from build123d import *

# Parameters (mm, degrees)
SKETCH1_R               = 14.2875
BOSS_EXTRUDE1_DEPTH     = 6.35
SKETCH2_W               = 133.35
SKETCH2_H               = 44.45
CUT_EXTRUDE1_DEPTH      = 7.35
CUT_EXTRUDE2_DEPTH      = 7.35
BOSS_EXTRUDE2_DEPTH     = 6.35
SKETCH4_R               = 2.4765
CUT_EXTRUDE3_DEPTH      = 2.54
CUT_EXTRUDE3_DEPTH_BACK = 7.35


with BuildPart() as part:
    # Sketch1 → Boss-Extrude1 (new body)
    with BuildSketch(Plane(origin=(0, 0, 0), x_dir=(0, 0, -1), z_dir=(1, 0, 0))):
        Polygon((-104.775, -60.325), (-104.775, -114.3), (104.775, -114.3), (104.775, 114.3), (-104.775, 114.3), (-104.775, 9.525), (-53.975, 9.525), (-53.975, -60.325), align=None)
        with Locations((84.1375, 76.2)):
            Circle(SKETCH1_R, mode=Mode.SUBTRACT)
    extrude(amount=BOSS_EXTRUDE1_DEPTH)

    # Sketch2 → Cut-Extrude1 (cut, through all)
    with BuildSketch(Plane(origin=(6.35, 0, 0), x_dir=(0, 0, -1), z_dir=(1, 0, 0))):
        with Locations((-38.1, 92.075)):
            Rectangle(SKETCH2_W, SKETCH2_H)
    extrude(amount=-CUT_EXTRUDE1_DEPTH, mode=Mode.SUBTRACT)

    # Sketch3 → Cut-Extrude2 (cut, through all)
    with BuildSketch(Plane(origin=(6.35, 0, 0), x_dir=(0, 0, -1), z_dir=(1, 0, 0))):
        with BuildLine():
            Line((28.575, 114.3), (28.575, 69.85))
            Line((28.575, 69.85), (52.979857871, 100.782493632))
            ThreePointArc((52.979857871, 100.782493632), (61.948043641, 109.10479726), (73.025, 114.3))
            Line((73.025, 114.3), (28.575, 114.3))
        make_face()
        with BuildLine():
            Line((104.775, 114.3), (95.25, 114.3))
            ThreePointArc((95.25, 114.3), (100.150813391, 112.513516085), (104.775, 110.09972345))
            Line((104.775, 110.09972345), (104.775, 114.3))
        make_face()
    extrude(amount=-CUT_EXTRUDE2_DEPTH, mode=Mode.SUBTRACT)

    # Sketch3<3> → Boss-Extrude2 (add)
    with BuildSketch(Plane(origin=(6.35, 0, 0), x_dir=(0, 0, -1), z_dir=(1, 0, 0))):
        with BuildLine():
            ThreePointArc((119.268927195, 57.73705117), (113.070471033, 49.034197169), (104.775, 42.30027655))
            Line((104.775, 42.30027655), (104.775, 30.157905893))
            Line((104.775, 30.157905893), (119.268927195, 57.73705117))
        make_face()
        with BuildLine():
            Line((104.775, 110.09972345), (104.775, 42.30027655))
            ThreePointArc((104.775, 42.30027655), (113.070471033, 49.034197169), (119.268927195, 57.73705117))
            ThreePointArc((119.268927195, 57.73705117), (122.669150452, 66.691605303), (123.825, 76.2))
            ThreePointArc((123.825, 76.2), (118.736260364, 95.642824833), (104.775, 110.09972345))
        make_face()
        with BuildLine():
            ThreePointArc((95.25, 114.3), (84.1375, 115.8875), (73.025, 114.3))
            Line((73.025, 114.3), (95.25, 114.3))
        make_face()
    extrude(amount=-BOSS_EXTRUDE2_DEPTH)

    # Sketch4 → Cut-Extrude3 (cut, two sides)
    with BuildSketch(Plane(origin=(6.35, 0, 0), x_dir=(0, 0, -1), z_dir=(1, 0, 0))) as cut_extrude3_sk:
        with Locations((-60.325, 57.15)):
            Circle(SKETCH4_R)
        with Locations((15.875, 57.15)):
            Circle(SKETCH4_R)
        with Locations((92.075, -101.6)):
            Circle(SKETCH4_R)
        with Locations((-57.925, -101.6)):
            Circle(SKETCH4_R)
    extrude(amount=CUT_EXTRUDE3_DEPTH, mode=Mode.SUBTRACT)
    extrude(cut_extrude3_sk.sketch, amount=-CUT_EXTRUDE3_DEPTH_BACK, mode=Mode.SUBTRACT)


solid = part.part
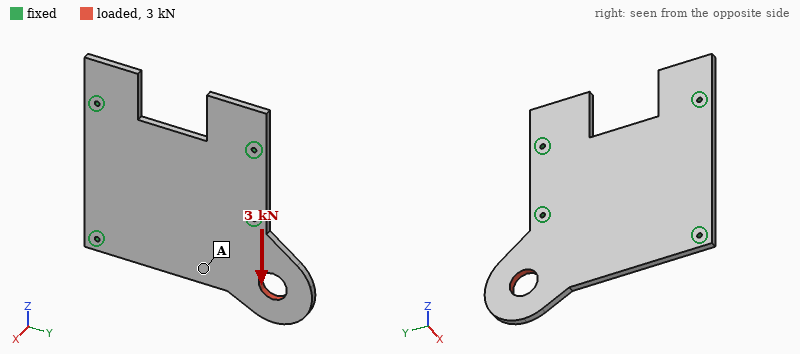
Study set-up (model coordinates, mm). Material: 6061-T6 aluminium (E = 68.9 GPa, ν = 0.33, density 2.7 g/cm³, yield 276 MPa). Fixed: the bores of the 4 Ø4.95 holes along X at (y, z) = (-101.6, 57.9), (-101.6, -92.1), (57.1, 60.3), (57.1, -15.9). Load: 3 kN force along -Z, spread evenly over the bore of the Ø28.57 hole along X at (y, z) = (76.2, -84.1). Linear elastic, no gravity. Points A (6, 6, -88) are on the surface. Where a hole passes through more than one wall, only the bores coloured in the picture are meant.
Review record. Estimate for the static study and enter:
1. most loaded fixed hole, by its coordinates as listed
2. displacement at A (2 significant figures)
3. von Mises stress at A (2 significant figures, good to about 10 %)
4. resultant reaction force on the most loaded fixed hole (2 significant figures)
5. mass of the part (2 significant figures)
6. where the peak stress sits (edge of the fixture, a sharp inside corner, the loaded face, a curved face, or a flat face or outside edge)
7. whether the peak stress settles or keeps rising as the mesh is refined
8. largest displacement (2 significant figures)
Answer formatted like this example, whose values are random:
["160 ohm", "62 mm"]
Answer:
["(57.1, -15.9)", "5.4 µm", "4.0 MPa", "2.7 kN", "650 g", "edge of the fixture", "keeps rising", "32 µm"]
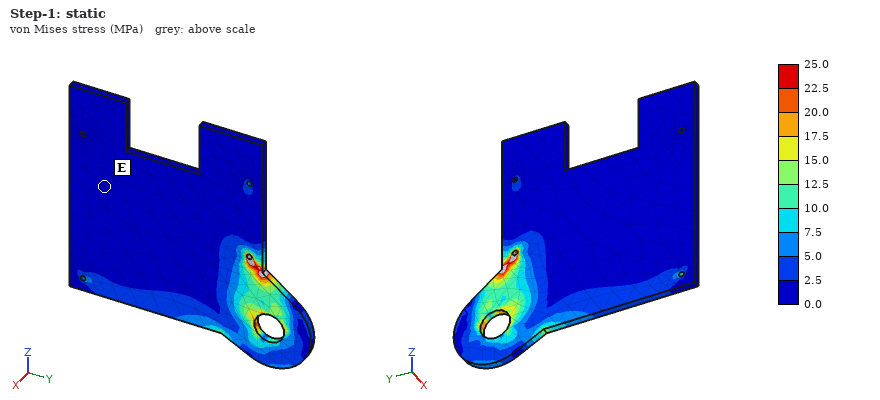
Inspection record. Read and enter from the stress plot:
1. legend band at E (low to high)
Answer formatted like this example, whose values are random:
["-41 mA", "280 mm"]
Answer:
["0.0 to 2.5 MPa"]
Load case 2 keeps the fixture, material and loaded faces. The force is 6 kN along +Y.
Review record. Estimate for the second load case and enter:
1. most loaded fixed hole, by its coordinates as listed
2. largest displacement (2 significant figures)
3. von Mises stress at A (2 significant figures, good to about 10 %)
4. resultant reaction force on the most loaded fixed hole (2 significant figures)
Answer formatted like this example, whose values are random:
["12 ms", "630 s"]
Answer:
["(57.1, -15.9)", "61 µm", "16 MPa", "2.9 kN"]
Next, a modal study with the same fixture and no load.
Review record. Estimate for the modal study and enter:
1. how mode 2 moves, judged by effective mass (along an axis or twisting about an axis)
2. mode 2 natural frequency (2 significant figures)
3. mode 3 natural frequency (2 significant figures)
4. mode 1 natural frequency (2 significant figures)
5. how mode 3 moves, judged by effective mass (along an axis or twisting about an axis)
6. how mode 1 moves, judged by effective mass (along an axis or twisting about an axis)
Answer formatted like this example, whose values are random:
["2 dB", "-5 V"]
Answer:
["along X", "830 Hz", "1200 Hz", "460 Hz", "along X", "along X"]
